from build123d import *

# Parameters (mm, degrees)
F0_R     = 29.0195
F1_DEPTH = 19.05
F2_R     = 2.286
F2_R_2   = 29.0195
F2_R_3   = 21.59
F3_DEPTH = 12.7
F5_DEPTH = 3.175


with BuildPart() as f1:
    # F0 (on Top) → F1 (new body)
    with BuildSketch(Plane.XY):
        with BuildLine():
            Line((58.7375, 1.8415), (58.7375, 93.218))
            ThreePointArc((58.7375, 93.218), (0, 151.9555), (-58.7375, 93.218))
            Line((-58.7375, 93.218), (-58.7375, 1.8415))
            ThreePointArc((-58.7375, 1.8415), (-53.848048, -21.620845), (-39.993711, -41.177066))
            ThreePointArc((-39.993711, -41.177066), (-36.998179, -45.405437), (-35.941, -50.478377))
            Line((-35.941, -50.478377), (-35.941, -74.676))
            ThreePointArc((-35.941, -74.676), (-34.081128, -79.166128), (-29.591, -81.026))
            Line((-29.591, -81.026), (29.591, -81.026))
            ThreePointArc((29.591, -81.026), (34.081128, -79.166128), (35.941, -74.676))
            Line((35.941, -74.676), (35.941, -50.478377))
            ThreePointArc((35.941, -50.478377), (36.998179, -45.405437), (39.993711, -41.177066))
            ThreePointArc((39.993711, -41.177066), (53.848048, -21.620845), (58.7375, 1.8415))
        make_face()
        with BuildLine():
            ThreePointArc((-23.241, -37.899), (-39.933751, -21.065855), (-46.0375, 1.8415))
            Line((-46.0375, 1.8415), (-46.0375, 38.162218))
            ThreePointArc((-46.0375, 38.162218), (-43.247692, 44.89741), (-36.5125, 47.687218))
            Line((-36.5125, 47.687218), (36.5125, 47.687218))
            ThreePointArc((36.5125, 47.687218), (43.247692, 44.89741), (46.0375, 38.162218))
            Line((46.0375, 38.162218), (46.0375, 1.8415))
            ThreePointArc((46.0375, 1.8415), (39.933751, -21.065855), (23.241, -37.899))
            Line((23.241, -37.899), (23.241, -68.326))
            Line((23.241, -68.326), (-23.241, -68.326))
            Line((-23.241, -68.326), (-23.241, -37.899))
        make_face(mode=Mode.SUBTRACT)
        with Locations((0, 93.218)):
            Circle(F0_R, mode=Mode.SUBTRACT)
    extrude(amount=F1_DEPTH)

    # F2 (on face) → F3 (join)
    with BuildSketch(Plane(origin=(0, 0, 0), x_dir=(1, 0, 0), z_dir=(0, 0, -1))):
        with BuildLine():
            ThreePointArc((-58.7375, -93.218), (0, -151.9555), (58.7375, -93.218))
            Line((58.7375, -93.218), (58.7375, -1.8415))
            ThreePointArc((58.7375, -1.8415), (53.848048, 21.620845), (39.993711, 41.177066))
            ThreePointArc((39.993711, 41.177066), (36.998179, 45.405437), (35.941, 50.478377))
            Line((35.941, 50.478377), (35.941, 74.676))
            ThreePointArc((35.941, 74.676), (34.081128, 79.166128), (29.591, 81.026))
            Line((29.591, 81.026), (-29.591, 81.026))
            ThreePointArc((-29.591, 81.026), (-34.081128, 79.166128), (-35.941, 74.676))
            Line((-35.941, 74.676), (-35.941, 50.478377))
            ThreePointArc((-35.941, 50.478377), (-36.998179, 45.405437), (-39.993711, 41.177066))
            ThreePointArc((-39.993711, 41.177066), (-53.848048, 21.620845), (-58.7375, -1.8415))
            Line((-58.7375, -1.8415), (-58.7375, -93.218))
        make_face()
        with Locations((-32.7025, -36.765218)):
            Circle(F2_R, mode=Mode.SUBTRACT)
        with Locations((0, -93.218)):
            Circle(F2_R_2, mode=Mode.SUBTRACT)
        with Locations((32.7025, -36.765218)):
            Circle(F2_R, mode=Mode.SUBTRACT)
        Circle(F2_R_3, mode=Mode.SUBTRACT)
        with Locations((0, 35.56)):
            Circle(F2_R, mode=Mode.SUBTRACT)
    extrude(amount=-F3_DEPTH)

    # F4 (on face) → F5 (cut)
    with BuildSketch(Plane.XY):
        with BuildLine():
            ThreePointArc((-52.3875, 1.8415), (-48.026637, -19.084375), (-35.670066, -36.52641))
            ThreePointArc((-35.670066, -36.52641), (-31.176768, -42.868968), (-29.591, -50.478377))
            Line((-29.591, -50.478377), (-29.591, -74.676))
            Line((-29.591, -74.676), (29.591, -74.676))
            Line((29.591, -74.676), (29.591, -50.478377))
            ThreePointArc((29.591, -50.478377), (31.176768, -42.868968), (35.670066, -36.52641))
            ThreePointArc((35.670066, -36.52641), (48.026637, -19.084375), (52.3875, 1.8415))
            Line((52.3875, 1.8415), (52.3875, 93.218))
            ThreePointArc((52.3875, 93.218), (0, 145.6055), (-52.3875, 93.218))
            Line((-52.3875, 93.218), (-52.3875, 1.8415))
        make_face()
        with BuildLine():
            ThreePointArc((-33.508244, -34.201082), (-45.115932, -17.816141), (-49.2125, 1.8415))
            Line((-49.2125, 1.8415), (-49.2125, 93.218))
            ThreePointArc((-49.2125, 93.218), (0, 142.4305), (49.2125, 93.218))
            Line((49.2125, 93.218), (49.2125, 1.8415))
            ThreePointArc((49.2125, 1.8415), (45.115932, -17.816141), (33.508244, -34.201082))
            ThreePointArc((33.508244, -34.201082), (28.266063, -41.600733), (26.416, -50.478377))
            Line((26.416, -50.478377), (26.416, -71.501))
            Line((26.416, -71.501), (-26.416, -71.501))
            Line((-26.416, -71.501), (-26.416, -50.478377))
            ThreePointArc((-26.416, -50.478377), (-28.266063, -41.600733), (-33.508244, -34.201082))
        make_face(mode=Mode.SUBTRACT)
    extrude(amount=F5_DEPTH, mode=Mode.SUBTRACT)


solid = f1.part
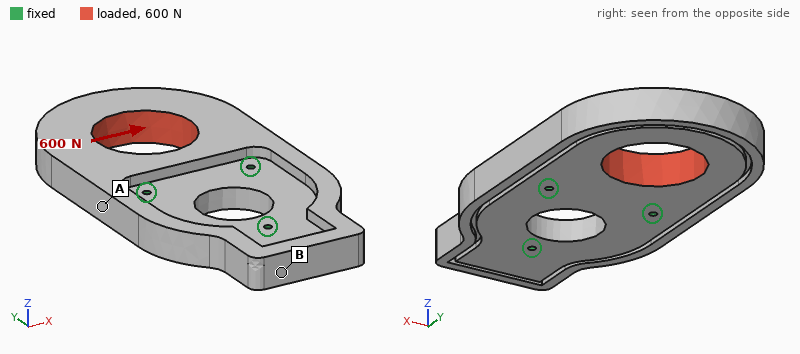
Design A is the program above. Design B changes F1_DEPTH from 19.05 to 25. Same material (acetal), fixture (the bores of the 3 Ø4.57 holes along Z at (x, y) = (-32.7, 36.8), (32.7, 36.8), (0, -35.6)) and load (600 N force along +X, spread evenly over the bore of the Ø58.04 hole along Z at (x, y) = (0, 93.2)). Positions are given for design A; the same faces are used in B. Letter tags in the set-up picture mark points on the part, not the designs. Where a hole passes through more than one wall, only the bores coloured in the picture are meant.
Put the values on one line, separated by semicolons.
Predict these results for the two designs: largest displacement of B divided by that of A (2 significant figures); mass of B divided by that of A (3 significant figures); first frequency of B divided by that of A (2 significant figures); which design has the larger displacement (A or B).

0.86; 1.23; 1.1; A
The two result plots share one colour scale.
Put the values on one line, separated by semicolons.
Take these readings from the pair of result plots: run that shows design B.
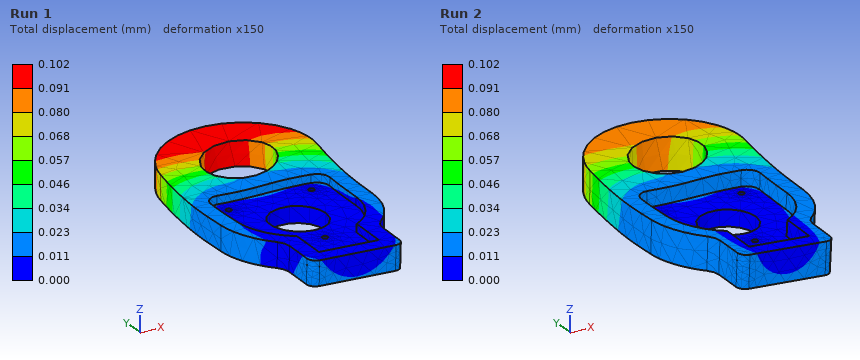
Run 2
